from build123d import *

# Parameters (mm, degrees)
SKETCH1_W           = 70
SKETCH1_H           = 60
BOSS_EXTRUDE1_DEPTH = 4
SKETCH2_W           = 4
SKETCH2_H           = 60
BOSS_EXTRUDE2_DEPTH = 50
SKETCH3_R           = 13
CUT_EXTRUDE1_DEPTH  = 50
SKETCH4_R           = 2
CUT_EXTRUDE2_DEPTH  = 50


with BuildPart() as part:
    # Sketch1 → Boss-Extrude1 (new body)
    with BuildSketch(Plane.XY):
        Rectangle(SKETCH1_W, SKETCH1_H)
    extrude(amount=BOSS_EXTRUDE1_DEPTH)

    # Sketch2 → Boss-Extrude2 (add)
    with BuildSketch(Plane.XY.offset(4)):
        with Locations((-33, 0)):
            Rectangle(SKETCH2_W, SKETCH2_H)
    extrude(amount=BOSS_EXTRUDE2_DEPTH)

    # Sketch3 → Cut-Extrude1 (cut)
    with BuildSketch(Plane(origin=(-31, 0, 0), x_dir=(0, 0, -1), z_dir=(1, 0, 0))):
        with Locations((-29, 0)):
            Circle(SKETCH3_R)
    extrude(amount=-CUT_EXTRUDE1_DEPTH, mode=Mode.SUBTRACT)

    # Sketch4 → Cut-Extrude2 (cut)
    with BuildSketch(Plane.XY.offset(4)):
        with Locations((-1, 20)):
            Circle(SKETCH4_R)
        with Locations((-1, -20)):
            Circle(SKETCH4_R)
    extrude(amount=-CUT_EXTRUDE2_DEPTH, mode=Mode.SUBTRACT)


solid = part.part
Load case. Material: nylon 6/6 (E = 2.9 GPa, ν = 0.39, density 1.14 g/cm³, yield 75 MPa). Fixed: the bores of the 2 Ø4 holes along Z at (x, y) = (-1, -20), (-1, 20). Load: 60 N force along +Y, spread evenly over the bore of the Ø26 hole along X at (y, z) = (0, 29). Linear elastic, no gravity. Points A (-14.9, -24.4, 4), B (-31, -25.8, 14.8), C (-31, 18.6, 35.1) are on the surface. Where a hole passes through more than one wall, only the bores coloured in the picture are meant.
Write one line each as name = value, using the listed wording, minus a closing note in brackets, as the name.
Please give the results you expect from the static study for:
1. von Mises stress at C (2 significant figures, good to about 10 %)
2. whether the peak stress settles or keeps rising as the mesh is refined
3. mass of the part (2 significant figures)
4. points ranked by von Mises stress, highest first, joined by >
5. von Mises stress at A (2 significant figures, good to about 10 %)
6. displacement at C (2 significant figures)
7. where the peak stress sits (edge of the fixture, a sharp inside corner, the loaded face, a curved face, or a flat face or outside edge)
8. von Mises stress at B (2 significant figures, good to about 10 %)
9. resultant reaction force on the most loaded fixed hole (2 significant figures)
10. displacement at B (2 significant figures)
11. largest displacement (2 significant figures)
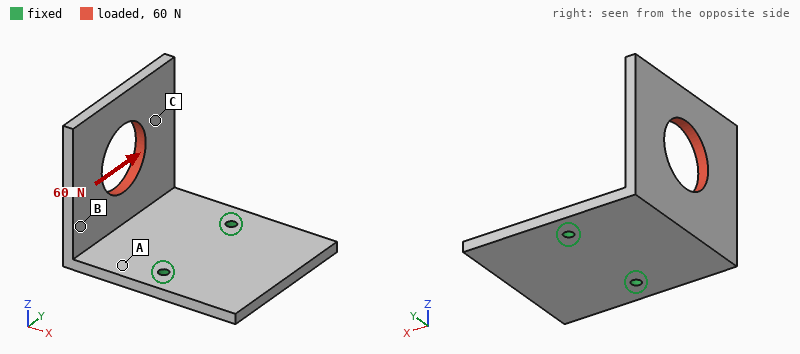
von Mises stress at C = 1.3 MPa
whether the peak stress settles or keeps rising as the mesh is refined = keeps rising
mass of the part = 30 g
points ranked by von Mises stress, highest first, joined by > = A > B > C
von Mises stress at A = 4.7 MPa
displacement at C = 0.68 mm
where the peak stress sits = edge of the fixture
von Mises stress at B = 2.9 MPa
resultant reaction force on the most loaded fixed hole = 67 N
displacement at B = 0.49 mm
largest displacement = 1.1 mm
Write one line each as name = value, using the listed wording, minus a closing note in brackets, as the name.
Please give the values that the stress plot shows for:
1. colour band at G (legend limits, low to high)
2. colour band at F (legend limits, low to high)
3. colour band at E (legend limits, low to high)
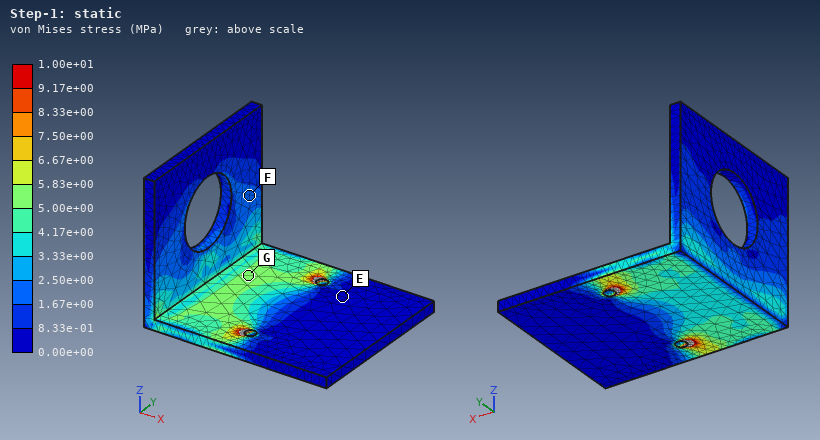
colour band at G = 5.00e+00 to 5.83e+00 MPa
colour band at F = 1.67e+00 to 2.50e+00 MPa
colour band at E = 0.00e+00 to 8.33e-01 MPa
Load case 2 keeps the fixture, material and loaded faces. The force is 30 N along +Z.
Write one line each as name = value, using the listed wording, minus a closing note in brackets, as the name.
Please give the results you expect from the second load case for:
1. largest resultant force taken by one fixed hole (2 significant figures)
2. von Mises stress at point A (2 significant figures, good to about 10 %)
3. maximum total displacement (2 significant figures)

largest resultant force taken by one fixed hole = 15 N
von Mises stress at point A = 3.4 MPa
maximum total displacement = 0.98 mm
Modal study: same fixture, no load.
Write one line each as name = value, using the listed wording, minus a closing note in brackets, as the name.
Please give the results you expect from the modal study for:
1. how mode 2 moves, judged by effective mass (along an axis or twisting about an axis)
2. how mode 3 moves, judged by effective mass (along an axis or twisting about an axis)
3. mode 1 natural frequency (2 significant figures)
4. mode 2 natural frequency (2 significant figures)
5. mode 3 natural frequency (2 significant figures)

how mode 2 moves, judged by effective mass = along Y
how mode 3 moves, judged by effective mass = along Z
mode 1 natural frequency = 200 Hz
mode 2 natural frequency = 380 Hz
mode 3 natural frequency = 560 Hz
